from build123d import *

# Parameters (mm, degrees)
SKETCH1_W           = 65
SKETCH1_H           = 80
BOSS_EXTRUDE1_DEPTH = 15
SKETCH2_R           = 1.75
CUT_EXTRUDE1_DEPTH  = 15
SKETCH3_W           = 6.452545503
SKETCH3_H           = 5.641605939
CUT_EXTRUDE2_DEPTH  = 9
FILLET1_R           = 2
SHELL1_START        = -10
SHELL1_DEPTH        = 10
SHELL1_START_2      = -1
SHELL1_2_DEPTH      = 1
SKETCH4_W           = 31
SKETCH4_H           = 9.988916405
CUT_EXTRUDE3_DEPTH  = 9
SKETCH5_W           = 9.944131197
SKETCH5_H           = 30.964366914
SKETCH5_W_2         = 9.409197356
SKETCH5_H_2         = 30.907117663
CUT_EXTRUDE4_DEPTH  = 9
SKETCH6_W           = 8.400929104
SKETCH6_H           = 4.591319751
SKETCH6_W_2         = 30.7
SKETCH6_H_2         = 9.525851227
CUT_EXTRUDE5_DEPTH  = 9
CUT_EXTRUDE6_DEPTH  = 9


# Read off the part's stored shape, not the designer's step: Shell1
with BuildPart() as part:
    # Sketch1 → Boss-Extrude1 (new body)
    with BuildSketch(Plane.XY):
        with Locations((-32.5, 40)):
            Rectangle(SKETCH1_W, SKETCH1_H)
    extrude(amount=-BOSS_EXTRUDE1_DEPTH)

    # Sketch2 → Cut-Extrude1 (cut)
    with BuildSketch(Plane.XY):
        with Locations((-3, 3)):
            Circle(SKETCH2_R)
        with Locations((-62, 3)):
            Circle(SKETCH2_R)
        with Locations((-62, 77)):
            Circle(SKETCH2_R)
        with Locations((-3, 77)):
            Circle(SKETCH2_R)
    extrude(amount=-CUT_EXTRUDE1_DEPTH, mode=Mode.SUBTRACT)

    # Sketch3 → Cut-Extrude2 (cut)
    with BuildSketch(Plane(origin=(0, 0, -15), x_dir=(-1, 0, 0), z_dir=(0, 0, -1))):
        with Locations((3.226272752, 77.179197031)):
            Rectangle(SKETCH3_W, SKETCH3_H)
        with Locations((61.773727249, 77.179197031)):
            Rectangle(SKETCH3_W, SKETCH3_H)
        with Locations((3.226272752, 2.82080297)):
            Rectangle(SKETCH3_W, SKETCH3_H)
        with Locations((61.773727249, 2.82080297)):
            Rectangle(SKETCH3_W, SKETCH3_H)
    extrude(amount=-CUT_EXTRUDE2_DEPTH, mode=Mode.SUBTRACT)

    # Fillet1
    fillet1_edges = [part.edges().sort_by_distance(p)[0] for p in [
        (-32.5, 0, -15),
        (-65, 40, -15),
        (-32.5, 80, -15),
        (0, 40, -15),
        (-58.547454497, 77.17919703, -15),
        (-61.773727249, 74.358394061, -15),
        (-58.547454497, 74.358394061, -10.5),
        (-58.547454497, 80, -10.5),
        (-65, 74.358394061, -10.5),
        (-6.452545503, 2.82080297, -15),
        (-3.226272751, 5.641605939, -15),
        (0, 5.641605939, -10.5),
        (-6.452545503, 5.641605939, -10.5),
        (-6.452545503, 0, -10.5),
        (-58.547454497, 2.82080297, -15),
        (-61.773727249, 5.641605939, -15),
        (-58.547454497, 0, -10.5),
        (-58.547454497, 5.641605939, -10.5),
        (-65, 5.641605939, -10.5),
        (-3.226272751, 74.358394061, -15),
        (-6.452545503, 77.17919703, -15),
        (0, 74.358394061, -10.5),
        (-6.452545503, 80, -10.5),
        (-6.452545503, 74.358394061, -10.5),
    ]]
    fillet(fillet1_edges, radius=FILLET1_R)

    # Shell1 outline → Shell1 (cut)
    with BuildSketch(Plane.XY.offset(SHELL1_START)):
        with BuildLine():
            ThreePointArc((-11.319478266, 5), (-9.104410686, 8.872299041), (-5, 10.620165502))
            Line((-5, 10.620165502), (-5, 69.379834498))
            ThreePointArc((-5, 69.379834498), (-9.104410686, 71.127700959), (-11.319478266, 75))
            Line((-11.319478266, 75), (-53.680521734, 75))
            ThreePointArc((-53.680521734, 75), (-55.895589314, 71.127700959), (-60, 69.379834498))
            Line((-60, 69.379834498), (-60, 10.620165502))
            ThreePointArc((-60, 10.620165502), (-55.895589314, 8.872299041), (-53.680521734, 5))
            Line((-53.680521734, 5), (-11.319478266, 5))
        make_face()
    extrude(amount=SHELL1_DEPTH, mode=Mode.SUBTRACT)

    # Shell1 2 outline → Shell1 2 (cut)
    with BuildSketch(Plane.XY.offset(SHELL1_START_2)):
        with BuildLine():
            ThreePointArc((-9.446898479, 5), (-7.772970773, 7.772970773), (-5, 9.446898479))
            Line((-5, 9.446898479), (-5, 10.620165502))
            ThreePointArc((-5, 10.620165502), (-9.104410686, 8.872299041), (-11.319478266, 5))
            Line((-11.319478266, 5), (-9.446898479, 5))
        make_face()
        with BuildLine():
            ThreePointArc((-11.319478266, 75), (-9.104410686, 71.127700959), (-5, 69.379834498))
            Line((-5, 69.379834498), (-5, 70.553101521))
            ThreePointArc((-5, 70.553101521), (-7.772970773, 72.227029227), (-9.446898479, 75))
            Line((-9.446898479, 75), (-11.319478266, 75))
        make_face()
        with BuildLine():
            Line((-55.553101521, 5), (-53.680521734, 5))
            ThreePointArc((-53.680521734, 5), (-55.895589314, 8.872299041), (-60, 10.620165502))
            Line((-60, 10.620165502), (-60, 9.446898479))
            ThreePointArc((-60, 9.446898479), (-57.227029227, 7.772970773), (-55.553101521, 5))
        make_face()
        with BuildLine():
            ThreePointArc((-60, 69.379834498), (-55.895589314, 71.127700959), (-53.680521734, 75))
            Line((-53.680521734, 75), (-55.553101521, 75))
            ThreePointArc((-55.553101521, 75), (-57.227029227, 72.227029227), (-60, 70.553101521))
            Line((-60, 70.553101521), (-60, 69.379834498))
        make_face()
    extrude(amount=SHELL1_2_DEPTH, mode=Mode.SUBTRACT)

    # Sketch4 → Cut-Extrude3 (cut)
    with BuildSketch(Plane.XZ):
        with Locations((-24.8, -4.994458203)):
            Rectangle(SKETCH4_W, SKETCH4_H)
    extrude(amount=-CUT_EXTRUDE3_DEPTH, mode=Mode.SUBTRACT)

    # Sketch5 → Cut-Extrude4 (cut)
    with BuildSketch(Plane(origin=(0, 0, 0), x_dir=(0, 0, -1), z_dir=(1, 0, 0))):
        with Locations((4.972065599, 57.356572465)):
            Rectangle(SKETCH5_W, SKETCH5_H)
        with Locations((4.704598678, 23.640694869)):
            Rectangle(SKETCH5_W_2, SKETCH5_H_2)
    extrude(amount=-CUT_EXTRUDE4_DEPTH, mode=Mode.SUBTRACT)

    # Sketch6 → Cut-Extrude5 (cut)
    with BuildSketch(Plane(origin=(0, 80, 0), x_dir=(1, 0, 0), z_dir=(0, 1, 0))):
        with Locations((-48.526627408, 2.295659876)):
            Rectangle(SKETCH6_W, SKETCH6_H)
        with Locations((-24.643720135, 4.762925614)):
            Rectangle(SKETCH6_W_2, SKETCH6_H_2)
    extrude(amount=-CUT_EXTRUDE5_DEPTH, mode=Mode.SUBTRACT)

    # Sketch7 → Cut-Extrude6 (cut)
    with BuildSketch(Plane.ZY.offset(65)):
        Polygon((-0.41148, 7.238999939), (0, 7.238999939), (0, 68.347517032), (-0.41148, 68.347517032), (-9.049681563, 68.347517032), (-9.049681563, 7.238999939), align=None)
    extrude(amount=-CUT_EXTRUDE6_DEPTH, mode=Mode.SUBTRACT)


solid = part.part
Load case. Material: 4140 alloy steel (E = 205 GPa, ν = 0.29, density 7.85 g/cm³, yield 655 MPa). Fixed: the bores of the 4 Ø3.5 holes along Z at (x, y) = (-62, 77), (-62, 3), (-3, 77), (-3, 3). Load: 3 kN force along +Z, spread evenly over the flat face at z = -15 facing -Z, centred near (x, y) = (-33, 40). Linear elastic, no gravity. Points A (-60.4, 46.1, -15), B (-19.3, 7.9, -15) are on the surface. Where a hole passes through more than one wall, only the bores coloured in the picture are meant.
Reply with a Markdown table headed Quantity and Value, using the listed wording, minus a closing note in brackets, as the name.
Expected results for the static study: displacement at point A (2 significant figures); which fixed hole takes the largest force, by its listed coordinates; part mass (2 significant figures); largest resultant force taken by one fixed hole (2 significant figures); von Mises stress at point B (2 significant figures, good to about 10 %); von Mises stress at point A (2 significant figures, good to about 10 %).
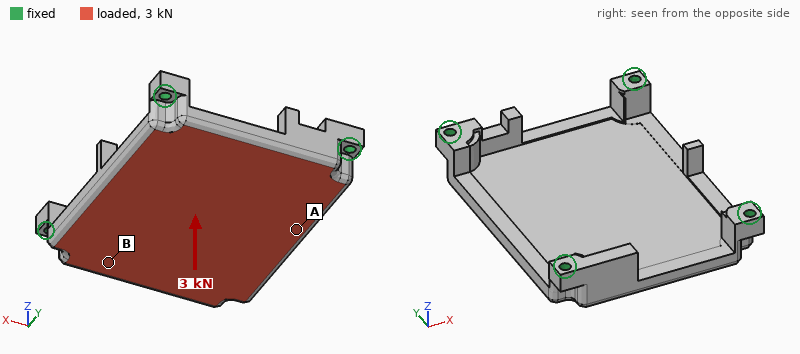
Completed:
| Quantity | Value |
|---|---|
| displacement at point A | 24 µm |
| which fixed hole takes the largest force, by its listed coordinates | (-62, 77) |
| part mass | 230 g |
| largest resultant force taken by one fixed hole | 1.4 kN |
| von Mises stress at point B | 20 MPa |
| von Mises stress at point A | 41 MPa |
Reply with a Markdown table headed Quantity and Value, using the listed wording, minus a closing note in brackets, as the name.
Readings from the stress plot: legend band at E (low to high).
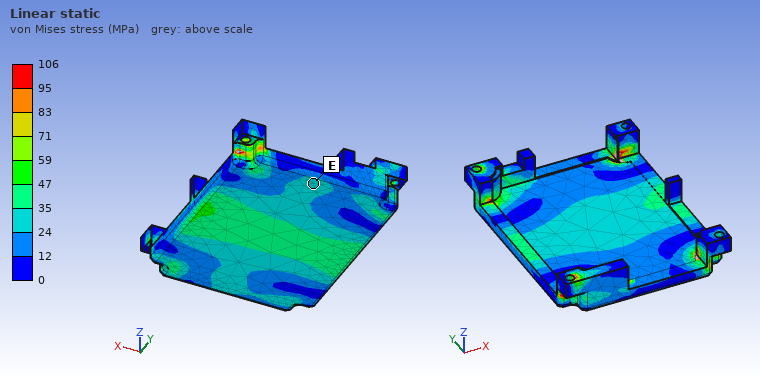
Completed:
| Quantity | Value |
|---|---|
| legend band at E | 24 to 35 MPa |
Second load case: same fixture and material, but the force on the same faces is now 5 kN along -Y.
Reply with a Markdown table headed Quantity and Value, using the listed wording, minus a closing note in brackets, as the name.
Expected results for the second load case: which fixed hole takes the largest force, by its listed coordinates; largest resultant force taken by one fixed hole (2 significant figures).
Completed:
| Quantity | Value |
|---|---|
| which fixed hole takes the largest force, by its listed coordinates | (-62, 77) |
| largest resultant force taken by one fixed hole | 1.7 kN |
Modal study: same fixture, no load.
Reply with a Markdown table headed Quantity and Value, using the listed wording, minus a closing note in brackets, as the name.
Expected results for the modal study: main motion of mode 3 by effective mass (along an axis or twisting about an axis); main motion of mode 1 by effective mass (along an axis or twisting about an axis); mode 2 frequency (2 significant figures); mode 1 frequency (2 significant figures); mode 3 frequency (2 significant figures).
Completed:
| Quantity | Value |
|---|---|
| main motion of mode 3 by effective mass | along Y |
| main motion of mode 1 by effective mass | along Z |
| mode 2 frequency | 5700 Hz |
| mode 1 frequency | 3800 Hz |
| mode 3 frequency | 6400 Hz |
